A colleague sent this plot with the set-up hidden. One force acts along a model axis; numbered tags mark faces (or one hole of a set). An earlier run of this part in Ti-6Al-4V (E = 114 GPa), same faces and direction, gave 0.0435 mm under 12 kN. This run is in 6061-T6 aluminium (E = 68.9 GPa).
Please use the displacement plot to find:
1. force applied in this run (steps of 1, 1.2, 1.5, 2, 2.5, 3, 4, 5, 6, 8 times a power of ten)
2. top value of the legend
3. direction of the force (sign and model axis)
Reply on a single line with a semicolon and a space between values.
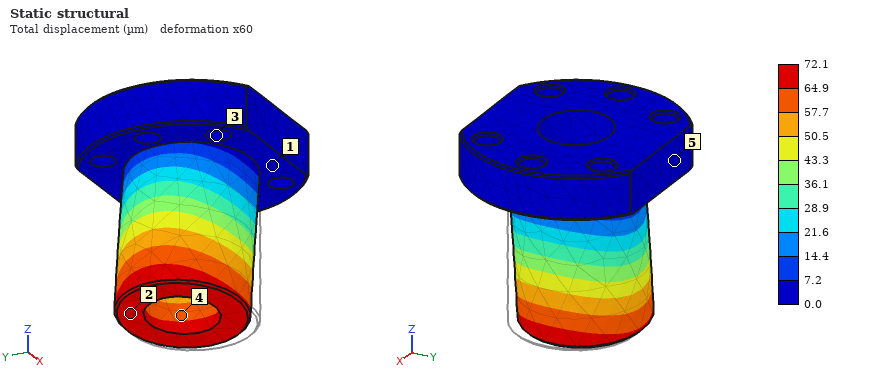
12 kN; 72.1 µm; -X
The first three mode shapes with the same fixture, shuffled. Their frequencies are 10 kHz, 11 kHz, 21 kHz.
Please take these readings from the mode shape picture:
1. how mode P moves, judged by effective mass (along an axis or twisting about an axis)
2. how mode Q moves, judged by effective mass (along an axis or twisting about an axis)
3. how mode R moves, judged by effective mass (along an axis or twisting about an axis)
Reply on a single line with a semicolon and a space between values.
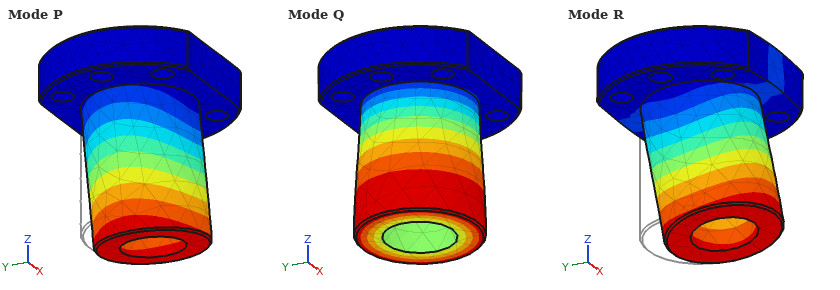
along X; twisting about Z; along Y
